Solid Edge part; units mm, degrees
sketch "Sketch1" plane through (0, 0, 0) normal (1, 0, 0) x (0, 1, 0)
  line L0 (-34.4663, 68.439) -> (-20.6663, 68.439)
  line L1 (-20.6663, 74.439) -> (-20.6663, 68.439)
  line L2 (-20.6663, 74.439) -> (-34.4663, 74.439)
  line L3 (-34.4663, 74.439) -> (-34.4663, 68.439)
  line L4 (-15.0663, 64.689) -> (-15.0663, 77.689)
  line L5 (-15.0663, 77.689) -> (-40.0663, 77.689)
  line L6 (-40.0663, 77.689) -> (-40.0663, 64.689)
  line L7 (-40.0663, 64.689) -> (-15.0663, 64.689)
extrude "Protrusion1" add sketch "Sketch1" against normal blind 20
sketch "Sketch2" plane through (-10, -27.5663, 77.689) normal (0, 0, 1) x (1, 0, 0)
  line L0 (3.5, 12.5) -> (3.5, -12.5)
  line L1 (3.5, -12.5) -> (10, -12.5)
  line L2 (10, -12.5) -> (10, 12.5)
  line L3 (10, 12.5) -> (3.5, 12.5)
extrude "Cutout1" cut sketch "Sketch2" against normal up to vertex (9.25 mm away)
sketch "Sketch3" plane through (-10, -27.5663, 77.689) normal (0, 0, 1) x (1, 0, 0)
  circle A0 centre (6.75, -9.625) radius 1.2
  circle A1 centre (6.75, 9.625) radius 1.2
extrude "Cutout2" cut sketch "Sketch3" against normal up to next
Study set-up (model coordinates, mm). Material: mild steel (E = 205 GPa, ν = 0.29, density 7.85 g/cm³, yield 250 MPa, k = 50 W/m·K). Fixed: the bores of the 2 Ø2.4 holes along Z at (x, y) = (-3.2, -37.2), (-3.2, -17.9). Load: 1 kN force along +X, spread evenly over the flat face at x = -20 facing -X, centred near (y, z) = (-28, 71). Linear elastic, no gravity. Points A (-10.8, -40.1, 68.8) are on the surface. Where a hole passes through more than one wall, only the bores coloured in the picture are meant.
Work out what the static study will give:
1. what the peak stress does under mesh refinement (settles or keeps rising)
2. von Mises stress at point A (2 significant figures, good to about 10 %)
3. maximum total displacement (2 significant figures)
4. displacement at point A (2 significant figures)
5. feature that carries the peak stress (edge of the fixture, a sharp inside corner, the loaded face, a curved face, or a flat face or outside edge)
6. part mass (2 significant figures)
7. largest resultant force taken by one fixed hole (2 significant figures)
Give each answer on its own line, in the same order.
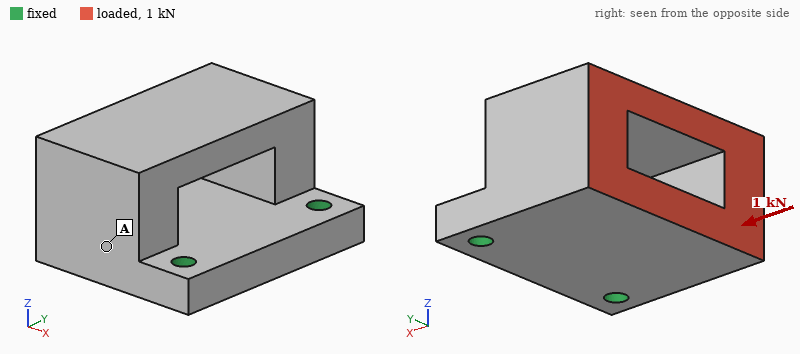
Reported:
keeps rising
24 MPa
27 µm
7.9 µm
edge of the fixture
30 g
500 N
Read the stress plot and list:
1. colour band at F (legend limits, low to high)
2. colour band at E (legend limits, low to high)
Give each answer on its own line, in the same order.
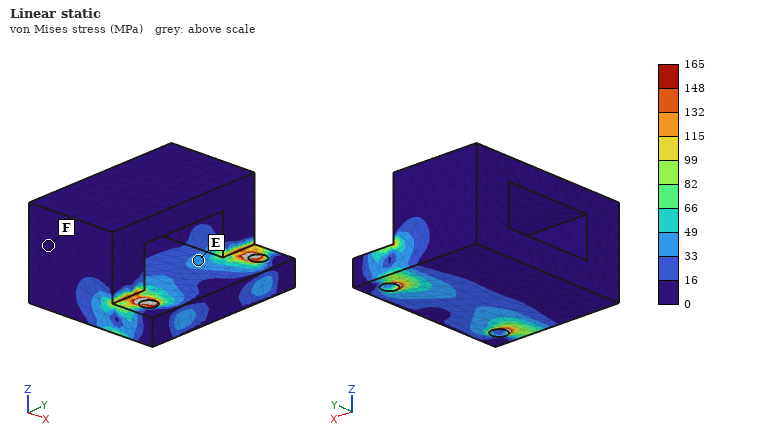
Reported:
0 to 16 MPa
33 to 49 MPa
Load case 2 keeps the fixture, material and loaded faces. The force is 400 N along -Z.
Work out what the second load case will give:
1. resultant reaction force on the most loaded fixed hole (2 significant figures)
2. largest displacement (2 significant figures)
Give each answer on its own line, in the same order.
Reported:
200 N
35 µm
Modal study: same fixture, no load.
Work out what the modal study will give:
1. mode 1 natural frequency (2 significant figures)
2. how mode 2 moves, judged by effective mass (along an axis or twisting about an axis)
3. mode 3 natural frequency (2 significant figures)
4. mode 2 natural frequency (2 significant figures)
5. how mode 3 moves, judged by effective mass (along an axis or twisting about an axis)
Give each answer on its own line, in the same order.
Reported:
5200 Hz
along Y
19 kHz
13 kHz
along Y
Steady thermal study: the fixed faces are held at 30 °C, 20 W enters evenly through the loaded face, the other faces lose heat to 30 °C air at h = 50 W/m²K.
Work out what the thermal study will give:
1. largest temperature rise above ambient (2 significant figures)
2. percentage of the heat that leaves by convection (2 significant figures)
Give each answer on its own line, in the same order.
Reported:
52 K
17 %
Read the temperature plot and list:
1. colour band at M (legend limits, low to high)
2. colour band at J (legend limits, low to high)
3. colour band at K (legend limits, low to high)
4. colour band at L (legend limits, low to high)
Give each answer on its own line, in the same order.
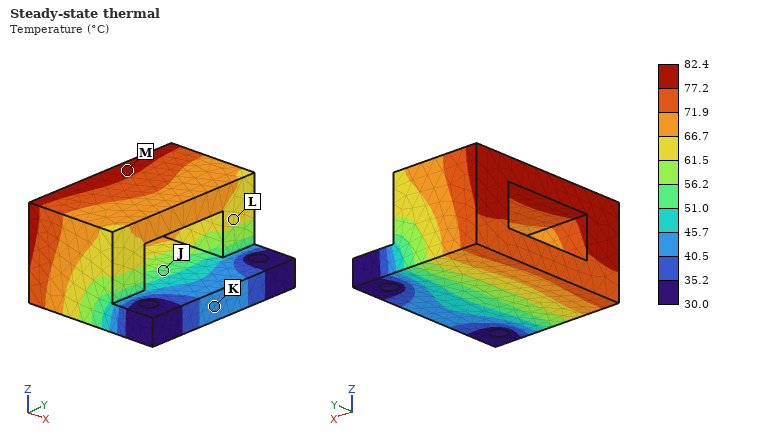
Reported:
77.2 to 82.4 °C
51.0 to 56.2 °C
40.5 to 45.7 °C
61.5 to 66.7 °C
